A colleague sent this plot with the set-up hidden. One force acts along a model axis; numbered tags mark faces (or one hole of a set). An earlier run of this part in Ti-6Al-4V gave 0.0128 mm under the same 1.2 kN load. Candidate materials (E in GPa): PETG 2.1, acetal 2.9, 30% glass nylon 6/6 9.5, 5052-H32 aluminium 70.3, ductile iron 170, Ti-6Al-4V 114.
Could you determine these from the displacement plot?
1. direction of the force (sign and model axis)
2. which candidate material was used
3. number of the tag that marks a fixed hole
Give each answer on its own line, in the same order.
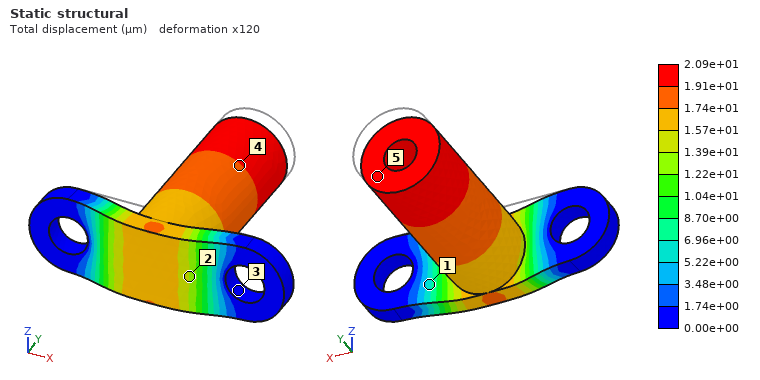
-Y
5052-H32 aluminium
3
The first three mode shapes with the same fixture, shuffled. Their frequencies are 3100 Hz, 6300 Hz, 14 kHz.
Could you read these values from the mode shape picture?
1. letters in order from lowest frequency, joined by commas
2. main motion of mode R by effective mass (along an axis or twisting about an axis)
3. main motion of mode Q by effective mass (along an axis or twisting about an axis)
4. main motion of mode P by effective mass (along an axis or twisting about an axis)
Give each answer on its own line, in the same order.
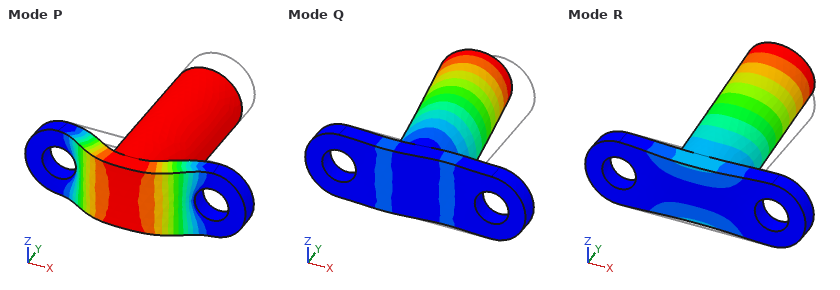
R, Q, P
along Z
along X
along Y
